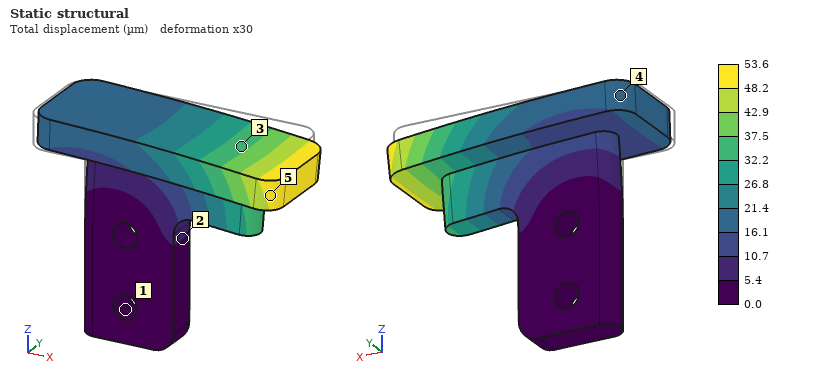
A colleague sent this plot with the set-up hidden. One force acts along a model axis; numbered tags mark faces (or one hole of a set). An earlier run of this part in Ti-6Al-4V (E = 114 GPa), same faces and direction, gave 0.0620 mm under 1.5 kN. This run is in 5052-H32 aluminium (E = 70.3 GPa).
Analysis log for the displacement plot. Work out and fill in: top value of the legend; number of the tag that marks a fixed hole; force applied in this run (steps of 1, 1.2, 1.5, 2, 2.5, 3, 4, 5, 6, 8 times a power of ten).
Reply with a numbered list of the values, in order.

1. 53.6 µm
2. 1
3. 800 N
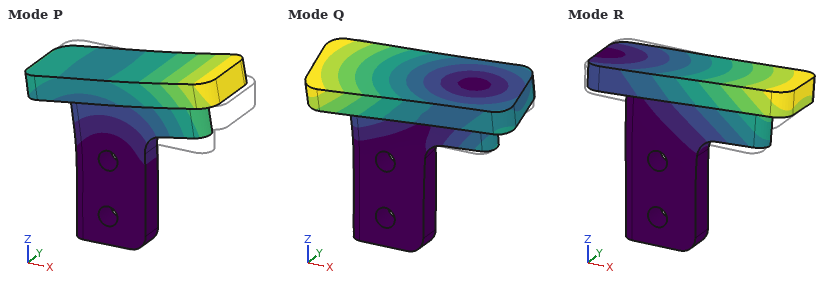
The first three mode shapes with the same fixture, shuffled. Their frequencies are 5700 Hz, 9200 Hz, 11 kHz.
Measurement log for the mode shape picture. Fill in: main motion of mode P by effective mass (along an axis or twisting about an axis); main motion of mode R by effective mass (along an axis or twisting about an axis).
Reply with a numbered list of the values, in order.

1. along X
2. along Y
